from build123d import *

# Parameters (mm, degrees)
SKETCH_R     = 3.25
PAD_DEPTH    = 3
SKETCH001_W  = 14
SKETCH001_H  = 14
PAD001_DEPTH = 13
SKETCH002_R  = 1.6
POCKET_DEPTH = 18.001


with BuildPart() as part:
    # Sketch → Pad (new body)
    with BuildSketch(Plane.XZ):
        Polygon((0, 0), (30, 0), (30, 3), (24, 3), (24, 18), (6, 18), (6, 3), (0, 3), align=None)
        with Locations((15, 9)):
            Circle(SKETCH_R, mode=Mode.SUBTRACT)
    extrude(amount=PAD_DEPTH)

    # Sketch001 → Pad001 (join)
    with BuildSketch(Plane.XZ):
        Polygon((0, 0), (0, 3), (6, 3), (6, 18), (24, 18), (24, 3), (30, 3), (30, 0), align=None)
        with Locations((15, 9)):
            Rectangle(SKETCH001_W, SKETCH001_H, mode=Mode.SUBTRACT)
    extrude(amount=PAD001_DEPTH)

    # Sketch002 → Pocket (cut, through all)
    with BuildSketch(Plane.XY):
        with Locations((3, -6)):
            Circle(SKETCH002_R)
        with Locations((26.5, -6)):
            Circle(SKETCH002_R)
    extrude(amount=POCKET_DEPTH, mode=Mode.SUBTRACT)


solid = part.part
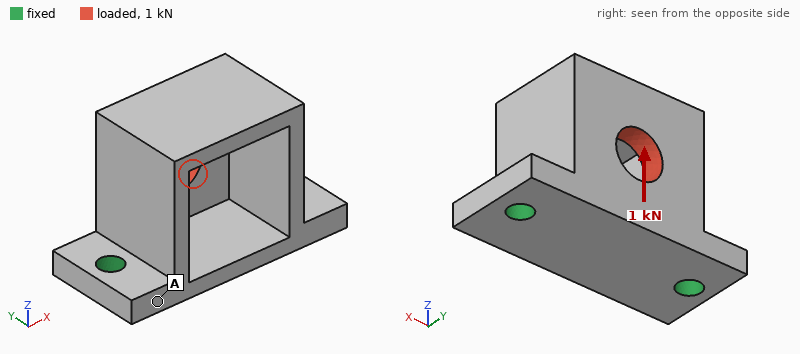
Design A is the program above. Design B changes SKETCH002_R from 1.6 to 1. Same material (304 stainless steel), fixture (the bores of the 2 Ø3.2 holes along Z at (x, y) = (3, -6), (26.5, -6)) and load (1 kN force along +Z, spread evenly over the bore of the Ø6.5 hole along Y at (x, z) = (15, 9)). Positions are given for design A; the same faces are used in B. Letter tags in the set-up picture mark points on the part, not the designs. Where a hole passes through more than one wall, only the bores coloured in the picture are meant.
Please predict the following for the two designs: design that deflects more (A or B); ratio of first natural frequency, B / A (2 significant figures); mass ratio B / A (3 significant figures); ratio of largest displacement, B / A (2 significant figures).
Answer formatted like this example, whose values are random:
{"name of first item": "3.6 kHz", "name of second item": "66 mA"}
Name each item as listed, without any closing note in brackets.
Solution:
{"design that deflects more": "B", "ratio of first natural frequency, B / A": "0.83", "mass ratio B / A": "1.01", "ratio of largest displacement, B / A": "1.5"}
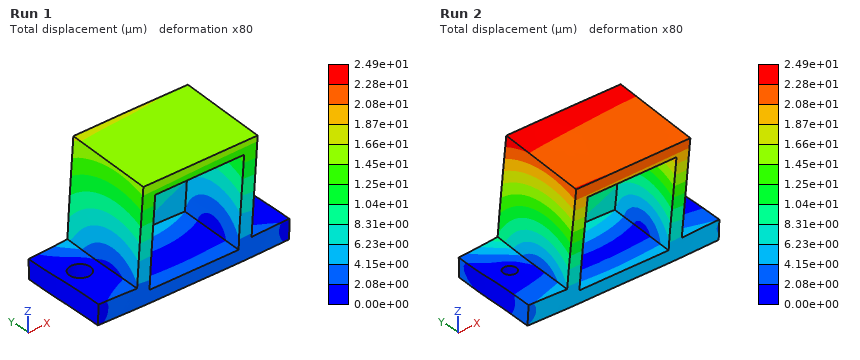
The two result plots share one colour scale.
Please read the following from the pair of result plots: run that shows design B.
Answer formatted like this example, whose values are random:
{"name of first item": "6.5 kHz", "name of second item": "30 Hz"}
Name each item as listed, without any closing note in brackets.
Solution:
{"run that shows design B": "Run 2"}
